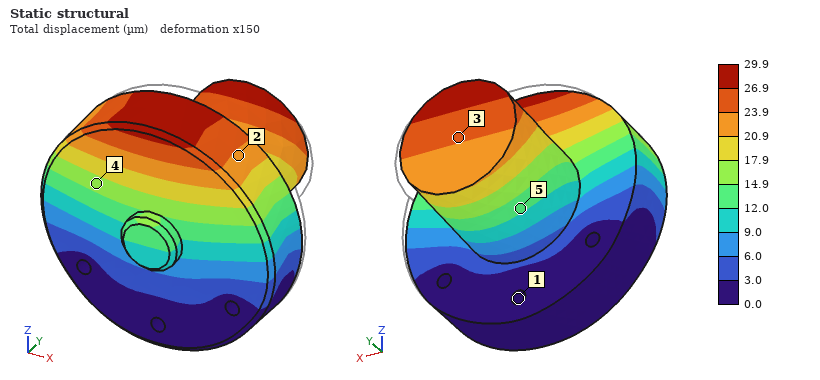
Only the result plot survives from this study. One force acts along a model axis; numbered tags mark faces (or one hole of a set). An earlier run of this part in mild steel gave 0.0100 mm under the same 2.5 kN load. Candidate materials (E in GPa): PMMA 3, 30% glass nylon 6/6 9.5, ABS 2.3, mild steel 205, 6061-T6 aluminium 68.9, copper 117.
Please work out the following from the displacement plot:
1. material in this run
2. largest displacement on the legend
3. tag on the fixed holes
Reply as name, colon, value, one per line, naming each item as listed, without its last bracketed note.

material in this run: 6061-T6 aluminium
largest displacement on the legend: 29.9 µm
tag on the fixed holes: 1
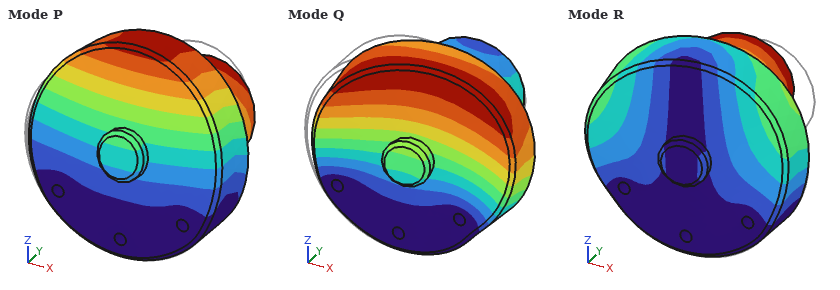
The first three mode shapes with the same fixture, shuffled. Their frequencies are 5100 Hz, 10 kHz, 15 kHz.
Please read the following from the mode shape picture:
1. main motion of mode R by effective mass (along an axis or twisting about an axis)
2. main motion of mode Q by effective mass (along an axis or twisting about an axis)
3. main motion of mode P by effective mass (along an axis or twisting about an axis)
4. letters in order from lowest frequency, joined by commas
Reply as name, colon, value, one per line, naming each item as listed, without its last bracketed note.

main motion of mode R by effective mass: along X
main motion of mode Q by effective mass: along X
main motion of mode P by effective mass: along Y
letters in order from lowest frequency, joined by commas: P, R, Q
